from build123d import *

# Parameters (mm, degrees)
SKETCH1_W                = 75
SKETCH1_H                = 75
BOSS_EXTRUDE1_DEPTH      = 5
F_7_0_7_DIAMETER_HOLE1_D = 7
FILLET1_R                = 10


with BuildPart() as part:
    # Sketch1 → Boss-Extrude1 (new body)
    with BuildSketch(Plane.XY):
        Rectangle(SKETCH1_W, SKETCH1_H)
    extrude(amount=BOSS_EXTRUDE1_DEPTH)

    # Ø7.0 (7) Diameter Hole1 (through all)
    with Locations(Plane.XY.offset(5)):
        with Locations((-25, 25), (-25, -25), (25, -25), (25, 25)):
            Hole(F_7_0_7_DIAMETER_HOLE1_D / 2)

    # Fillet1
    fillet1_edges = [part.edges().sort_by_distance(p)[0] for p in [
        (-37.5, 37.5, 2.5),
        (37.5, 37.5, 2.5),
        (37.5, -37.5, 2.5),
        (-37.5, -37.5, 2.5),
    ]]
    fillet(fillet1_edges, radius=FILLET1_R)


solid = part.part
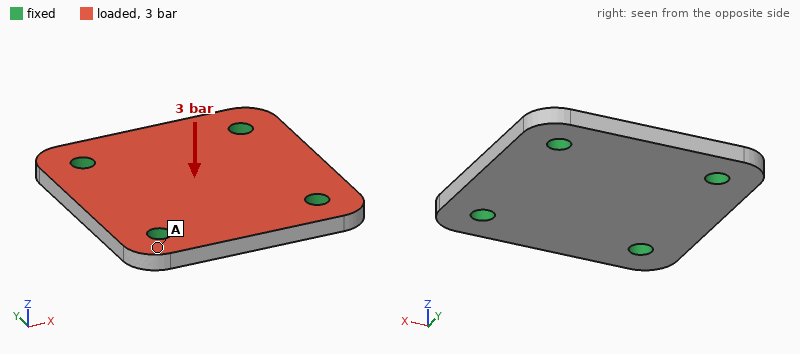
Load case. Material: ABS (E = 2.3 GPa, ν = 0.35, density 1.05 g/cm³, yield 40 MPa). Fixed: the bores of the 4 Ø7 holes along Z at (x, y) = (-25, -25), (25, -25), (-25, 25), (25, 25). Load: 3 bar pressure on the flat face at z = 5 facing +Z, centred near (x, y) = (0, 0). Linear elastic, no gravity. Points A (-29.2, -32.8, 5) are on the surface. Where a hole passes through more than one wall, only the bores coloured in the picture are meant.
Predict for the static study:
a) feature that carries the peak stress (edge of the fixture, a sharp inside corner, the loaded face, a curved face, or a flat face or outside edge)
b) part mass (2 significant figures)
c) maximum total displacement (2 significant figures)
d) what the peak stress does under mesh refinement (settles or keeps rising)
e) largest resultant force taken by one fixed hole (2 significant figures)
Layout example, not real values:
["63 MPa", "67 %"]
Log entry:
["edge of the fixture", "28 g", "0.38 mm", "keeps rising", "400 N"]
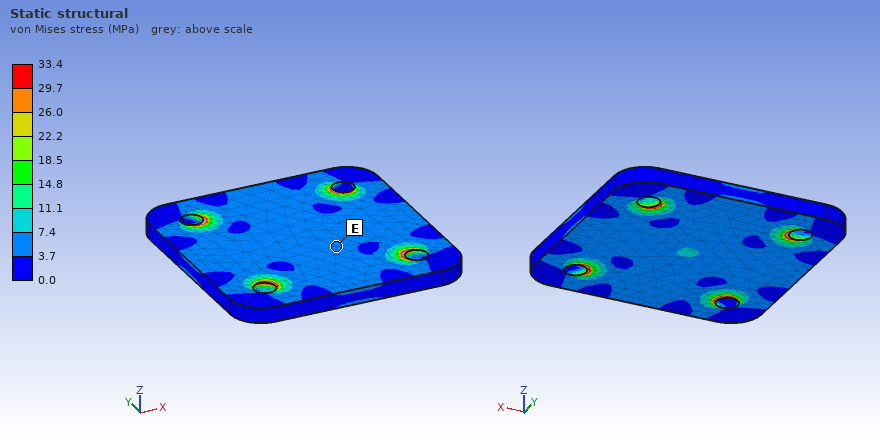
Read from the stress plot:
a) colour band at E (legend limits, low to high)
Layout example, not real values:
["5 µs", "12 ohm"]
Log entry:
["3.7 to 7.4 MPa"]
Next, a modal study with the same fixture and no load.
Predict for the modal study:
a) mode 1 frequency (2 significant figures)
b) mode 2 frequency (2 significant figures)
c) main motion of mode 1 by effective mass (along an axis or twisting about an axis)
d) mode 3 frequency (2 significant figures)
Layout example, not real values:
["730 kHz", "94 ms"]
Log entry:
["2400 Hz", "3300 Hz", "along Z", "3300 Hz"]
